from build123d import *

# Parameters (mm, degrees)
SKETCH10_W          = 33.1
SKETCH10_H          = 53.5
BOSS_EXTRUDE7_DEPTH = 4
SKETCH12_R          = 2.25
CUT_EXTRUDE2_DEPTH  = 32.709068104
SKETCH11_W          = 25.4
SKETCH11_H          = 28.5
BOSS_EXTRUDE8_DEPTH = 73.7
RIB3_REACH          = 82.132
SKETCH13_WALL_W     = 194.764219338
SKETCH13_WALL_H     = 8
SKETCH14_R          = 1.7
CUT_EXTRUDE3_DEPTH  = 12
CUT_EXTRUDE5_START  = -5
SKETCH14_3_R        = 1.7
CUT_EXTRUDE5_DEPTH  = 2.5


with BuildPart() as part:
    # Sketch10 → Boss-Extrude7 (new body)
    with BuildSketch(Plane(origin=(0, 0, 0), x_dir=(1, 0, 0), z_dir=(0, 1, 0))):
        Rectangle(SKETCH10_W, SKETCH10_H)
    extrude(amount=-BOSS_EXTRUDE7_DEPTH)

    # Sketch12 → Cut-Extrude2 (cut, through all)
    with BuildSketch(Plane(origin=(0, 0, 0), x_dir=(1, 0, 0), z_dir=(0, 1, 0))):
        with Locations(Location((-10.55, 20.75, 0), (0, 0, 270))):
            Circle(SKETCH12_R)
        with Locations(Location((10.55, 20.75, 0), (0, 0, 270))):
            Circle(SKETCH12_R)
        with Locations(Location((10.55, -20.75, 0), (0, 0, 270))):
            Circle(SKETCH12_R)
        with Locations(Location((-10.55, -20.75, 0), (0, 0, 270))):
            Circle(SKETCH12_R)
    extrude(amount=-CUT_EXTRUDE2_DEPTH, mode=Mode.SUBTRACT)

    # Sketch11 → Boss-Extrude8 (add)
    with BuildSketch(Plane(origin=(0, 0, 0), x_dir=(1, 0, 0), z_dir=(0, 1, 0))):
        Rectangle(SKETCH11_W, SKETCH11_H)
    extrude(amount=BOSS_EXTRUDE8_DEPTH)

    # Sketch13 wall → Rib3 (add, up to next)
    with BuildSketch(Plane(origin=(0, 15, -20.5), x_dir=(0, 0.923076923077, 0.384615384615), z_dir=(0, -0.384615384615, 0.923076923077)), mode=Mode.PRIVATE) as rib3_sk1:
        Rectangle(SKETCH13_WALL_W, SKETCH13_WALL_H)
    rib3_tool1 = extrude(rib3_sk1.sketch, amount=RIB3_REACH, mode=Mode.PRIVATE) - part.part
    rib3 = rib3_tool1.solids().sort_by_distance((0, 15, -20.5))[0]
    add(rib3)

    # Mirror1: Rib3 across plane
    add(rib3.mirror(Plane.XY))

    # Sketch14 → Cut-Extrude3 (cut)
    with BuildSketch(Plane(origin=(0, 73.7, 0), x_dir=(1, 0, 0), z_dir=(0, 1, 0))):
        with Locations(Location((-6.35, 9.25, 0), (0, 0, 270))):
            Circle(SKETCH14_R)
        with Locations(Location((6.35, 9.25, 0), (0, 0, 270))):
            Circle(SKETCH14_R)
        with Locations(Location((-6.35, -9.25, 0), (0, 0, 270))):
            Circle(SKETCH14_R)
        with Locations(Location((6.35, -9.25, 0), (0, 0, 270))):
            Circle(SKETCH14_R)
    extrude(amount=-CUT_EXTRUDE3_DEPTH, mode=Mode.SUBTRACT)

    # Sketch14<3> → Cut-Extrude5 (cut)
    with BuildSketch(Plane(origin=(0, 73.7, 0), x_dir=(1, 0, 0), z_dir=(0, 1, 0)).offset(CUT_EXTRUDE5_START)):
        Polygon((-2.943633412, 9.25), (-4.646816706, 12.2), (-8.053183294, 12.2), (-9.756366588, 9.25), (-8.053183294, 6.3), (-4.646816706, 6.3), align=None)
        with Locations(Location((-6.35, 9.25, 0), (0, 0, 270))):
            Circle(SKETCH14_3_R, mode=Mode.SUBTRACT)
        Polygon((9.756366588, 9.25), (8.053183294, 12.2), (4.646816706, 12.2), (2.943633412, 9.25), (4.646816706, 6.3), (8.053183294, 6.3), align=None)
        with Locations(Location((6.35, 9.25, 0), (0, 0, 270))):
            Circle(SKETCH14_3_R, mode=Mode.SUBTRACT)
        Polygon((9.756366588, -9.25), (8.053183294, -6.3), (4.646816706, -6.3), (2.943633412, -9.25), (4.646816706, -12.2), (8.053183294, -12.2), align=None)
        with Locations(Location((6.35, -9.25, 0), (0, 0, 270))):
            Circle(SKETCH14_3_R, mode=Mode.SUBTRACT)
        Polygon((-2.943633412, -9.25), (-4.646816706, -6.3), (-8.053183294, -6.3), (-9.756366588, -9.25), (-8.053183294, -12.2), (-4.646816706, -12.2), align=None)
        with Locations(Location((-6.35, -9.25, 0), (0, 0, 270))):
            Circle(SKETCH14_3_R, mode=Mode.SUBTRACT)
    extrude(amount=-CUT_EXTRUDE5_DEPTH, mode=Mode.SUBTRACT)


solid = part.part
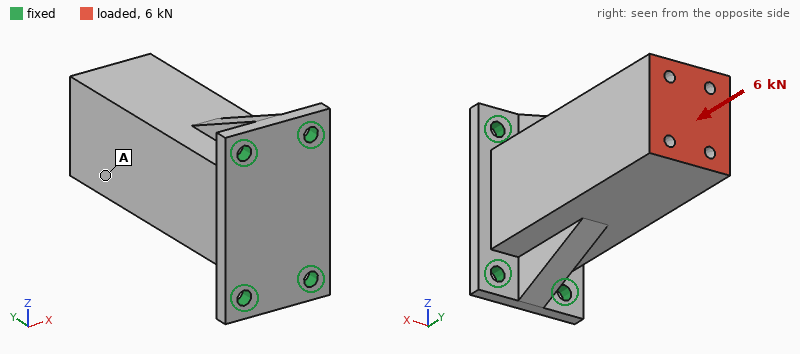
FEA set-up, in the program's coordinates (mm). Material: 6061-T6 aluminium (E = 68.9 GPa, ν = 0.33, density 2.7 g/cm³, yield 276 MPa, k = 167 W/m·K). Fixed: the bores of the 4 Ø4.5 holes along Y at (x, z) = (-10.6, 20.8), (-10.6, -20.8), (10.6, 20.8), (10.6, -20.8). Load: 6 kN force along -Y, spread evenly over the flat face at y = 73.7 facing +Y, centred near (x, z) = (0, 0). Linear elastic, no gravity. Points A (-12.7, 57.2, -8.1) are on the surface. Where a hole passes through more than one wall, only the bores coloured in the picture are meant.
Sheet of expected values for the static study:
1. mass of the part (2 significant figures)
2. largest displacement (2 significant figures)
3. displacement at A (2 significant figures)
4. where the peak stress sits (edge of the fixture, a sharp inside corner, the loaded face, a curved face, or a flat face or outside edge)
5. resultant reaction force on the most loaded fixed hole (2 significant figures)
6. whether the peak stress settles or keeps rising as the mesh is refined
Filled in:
170 g
23 µm
20 µm
edge of the fixture
1.6 kN
keeps rising
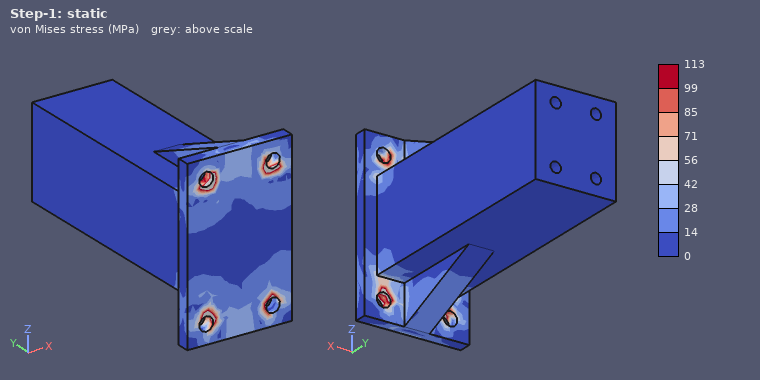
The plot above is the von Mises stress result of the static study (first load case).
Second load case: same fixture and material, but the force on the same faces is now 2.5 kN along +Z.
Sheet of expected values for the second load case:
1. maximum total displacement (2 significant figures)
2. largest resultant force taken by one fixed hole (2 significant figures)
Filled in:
0.16 mm
2.6 kN
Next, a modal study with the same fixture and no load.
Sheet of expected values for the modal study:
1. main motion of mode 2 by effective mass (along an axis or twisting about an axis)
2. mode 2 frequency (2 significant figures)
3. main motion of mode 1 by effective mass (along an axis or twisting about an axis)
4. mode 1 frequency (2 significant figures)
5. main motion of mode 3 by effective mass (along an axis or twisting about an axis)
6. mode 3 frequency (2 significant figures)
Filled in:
along Z
3100 Hz
along X
1600 Hz
along Y
7700 Hz
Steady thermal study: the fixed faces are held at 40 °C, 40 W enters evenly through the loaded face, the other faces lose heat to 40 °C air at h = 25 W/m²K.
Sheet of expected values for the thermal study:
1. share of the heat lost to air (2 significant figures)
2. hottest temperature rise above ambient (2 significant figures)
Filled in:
11 %
29 K
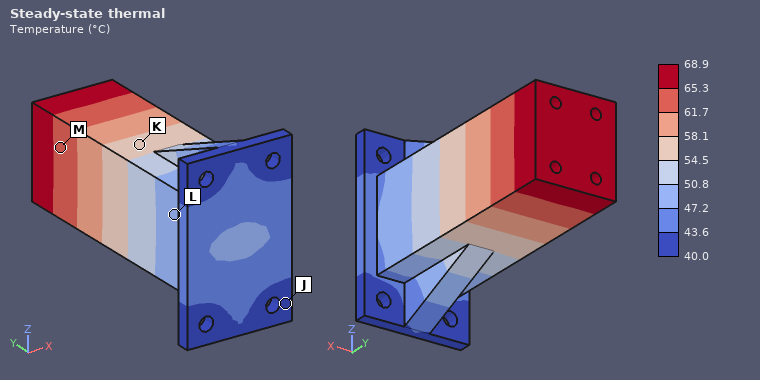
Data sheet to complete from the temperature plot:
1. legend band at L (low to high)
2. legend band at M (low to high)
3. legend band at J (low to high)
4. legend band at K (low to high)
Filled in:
47.2 to 50.8 °C
61.7 to 65.3 °C
40.0 to 43.6 °C
54.5 to 58.1 °C
